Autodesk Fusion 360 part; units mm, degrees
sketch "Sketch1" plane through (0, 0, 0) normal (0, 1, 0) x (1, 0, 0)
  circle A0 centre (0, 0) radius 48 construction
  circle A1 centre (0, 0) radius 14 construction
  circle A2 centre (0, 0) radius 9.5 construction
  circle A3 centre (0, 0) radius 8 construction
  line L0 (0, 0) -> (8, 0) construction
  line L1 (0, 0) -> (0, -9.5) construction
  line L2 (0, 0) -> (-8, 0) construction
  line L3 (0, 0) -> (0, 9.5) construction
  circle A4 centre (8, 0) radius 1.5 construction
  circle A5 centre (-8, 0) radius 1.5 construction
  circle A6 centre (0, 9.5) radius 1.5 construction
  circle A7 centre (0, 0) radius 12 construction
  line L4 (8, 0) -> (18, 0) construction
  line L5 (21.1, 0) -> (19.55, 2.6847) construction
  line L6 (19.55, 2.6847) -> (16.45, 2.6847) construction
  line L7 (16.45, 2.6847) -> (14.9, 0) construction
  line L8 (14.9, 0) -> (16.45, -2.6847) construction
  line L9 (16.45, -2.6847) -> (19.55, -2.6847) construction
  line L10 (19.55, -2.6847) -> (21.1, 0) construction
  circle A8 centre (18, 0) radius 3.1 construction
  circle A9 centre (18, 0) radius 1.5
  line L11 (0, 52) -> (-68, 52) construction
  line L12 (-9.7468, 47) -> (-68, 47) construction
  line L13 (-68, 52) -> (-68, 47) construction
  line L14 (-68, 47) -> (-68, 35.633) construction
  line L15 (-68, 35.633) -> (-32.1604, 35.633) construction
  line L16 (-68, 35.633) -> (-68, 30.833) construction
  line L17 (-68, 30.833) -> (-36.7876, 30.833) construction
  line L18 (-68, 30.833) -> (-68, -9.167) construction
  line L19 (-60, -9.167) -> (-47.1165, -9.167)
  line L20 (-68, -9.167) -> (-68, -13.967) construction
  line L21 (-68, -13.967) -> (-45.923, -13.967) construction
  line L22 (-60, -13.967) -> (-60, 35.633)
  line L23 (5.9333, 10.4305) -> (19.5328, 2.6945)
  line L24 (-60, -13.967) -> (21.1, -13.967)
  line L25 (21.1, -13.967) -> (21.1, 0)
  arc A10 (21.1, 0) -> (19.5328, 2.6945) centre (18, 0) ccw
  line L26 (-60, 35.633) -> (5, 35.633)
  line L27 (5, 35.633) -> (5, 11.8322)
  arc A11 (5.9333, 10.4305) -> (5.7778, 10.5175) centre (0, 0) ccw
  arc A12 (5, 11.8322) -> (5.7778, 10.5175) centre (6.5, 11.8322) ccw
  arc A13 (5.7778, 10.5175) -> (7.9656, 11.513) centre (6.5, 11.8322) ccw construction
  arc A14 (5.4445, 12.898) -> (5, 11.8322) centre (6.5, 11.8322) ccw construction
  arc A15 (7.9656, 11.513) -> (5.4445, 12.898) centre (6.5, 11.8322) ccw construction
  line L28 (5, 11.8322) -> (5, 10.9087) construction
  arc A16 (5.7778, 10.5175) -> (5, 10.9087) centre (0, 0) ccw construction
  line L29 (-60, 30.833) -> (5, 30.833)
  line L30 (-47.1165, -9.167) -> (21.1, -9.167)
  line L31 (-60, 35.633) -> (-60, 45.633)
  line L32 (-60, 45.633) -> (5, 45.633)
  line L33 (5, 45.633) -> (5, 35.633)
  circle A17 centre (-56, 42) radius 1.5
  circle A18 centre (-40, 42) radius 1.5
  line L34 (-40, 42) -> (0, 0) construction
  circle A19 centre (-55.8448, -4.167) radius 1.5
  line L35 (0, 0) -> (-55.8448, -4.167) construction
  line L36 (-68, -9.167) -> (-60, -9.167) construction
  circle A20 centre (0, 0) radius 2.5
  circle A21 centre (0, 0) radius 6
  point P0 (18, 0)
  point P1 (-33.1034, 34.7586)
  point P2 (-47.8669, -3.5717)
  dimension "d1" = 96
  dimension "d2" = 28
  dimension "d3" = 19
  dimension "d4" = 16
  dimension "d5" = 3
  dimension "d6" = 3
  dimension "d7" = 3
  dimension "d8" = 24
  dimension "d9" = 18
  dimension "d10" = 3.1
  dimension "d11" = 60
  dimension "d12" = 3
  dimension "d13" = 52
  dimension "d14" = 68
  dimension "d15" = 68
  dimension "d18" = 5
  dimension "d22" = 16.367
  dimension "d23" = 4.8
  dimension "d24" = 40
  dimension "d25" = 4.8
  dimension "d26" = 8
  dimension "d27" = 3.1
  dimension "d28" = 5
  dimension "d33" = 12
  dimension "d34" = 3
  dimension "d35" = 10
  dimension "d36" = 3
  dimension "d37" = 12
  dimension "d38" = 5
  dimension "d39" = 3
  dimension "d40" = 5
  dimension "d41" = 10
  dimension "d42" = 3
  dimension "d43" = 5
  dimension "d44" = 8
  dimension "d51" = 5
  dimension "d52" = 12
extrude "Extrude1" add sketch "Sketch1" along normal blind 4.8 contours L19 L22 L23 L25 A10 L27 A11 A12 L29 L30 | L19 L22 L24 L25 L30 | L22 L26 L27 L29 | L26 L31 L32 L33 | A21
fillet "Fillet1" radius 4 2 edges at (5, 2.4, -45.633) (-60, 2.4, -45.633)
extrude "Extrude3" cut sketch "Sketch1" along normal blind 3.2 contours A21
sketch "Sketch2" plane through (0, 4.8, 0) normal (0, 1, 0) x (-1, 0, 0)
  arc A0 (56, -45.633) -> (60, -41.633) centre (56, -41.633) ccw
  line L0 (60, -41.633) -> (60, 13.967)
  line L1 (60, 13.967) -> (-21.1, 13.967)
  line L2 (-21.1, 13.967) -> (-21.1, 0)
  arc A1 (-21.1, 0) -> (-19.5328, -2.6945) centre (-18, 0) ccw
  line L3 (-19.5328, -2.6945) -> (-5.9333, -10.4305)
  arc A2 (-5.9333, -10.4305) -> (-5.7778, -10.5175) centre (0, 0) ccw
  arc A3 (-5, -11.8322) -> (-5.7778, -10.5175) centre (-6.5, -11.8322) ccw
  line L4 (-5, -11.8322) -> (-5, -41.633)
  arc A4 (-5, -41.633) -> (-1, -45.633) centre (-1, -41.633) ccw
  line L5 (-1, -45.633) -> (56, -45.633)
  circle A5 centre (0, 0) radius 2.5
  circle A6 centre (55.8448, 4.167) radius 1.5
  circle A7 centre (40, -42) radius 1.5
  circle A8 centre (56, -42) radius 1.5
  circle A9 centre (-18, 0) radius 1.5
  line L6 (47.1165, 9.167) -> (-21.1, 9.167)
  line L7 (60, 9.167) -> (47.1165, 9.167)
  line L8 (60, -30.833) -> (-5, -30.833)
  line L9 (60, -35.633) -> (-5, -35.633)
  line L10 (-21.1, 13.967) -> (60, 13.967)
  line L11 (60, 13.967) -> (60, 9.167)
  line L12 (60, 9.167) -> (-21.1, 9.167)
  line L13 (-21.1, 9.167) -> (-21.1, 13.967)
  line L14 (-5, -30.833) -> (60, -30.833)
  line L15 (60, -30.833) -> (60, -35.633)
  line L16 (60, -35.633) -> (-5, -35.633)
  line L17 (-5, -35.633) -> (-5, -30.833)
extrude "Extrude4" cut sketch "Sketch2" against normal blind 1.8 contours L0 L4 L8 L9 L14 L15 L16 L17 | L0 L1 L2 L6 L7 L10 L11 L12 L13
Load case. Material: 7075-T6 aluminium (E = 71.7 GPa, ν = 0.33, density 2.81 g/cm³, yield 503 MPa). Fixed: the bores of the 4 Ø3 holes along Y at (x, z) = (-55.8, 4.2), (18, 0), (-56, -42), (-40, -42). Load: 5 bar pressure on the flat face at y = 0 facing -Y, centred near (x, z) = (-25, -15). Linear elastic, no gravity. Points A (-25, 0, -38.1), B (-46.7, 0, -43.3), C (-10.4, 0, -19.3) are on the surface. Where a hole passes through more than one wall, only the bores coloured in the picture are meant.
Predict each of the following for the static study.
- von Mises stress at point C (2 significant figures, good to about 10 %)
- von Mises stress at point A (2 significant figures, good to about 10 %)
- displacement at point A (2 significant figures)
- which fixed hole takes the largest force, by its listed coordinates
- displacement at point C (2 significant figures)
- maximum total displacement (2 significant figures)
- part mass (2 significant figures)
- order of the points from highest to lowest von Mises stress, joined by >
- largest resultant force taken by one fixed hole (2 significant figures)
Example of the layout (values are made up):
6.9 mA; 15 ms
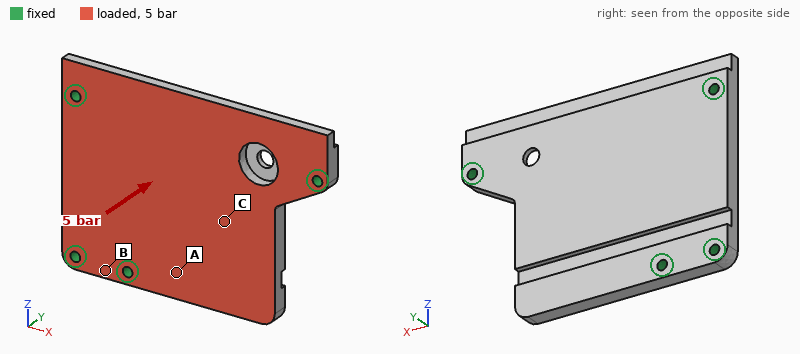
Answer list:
40 MPa; 22 MPa; 0.058 mm; (-40, -42); 0.10 mm; 0.19 mm; 52 g; C > A > B; 820 N
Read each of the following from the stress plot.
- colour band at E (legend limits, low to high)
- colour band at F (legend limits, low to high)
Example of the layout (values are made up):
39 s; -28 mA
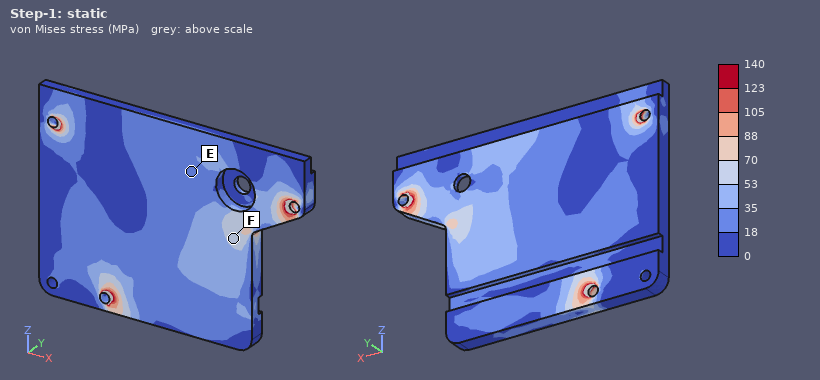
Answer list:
18 to 35 MPa; 53 to 70 MPa
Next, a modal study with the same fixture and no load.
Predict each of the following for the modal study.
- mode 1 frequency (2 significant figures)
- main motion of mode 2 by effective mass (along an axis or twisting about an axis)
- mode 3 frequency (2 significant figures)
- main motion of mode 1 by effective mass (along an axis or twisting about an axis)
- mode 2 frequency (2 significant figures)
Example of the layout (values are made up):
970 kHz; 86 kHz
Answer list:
3000 Hz; along Y; 8400 Hz; along Y; 4200 Hz
